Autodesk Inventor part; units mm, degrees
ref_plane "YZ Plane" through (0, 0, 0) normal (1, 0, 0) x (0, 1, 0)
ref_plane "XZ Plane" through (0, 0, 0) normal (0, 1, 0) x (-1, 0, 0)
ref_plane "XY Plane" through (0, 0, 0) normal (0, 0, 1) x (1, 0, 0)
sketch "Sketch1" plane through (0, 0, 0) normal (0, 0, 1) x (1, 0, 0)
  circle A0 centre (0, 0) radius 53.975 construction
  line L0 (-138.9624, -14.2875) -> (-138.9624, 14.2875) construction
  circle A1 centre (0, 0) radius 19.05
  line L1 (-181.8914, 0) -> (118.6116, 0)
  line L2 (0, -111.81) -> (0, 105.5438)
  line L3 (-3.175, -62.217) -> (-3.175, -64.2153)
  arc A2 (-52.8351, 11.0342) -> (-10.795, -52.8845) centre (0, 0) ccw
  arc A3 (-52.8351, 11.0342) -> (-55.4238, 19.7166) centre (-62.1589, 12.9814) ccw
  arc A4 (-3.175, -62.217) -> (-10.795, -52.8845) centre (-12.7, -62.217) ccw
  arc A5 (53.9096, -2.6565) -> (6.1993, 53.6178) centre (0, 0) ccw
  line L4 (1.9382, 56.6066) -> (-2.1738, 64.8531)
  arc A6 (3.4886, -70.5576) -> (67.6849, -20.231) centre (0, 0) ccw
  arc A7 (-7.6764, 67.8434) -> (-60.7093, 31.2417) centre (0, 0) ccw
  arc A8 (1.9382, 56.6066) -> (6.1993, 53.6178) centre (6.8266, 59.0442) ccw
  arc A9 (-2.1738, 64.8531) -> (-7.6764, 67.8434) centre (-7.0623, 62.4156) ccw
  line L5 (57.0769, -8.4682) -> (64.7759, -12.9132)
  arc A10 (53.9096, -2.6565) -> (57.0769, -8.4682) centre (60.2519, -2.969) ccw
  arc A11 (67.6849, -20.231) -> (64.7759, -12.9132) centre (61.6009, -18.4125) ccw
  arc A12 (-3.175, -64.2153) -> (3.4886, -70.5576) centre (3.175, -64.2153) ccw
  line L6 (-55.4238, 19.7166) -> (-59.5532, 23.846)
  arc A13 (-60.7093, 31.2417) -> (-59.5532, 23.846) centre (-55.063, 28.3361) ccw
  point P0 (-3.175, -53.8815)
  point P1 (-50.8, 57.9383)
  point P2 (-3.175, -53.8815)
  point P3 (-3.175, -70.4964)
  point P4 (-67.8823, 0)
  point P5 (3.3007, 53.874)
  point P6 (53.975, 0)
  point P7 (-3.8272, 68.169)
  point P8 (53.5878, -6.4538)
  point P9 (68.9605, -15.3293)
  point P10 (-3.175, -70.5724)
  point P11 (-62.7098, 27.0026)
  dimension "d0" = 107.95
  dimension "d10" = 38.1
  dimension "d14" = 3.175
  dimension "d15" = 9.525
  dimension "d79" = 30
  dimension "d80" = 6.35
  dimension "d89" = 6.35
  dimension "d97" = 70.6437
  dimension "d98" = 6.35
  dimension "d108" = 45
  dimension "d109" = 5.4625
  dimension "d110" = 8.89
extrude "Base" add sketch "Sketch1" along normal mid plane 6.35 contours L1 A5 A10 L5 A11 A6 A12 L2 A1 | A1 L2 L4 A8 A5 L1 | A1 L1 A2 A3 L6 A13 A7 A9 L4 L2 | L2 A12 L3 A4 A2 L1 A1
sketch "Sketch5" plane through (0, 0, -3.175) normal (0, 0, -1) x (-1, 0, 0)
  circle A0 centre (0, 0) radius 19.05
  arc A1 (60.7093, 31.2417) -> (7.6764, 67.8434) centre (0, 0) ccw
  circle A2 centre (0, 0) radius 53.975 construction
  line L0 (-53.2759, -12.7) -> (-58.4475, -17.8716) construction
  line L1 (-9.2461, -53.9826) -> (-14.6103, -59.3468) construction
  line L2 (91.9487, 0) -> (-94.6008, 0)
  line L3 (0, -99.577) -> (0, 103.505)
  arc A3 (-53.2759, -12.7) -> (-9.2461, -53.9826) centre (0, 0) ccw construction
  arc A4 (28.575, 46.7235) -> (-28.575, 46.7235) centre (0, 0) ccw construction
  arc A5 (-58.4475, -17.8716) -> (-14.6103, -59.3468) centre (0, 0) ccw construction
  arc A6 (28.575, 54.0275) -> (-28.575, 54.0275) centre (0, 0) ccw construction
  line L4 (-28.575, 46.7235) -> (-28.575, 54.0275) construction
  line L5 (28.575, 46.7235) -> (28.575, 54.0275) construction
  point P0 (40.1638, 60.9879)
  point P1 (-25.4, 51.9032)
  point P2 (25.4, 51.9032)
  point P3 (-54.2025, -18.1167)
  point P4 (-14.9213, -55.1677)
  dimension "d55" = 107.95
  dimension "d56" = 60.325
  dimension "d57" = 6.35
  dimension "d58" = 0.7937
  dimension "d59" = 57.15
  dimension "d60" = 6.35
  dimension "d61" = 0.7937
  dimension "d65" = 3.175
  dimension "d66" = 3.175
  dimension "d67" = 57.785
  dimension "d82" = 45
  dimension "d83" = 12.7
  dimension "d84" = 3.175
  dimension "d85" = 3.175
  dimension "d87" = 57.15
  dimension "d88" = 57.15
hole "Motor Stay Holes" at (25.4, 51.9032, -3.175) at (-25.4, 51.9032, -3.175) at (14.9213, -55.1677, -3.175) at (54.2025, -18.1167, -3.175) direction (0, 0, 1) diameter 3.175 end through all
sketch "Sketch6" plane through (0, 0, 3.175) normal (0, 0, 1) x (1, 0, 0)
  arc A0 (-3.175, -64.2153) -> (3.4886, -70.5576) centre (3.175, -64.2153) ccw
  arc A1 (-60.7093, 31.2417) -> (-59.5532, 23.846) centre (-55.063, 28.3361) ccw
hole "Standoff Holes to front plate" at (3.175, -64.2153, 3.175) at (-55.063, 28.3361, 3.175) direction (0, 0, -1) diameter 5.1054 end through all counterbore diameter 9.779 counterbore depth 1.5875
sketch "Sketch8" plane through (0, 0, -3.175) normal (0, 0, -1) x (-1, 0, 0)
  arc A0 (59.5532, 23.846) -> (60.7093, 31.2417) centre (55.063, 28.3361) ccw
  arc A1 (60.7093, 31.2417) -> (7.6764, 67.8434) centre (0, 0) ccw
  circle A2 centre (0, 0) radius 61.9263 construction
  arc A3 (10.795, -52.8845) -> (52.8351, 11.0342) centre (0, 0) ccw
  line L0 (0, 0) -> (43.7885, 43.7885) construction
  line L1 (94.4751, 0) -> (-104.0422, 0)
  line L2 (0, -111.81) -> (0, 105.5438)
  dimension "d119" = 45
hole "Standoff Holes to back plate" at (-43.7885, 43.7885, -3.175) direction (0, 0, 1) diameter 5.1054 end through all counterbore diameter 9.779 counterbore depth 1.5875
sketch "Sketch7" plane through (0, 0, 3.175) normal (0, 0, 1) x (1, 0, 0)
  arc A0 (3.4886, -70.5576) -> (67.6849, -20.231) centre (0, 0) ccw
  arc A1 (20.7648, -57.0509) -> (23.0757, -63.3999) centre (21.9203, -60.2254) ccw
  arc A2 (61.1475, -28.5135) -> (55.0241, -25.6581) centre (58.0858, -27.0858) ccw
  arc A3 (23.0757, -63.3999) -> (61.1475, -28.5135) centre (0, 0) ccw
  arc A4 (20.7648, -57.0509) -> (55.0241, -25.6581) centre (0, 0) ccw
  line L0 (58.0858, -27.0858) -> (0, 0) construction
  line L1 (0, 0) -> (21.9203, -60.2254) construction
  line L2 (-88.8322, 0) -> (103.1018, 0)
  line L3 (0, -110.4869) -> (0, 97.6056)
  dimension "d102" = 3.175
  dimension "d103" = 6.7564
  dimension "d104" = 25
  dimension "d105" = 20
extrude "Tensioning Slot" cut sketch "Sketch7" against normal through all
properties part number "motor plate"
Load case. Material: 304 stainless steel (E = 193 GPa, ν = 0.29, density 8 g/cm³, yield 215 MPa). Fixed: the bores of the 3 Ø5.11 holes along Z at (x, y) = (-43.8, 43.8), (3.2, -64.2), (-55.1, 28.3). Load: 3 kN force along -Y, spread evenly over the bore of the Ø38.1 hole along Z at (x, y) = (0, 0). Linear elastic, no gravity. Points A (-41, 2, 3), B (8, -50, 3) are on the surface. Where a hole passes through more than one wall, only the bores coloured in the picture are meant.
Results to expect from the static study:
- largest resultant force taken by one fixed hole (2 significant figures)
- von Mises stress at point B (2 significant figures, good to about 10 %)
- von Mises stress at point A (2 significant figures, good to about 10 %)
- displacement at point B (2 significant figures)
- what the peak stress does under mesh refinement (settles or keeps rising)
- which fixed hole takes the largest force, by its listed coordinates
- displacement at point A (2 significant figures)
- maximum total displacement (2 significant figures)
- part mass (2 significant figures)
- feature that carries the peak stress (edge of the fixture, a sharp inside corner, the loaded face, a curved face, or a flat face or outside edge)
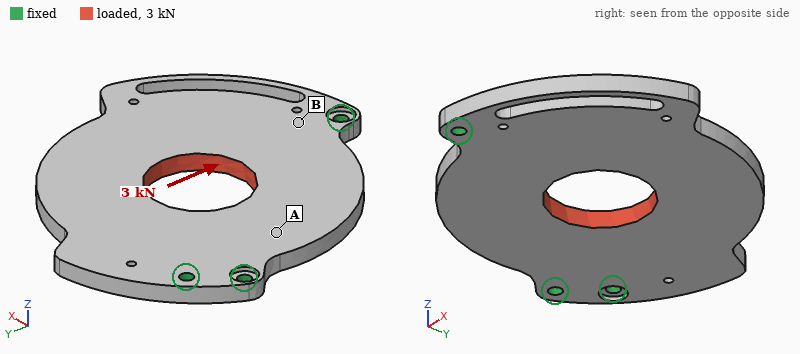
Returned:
1.7 kN
9.7 MPa
5.0 MPa
1.9 µm
keeps rising
(3.2, -64.2)
1.9 µm
6.1 µm
510 g
edge of the fixture
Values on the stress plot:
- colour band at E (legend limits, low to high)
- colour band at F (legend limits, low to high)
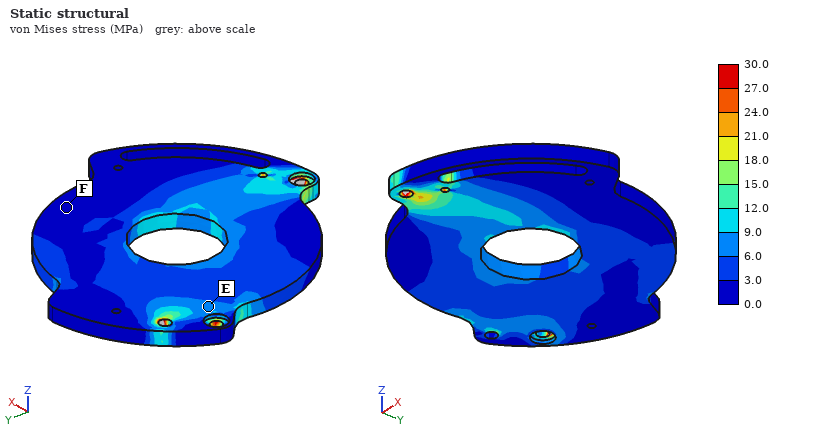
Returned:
6.0 to 9.0 MPa
0.0 to 3.0 MPa
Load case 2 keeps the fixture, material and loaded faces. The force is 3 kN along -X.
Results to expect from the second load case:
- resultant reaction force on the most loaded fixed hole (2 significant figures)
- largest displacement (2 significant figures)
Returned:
1.1 kN
4.0 µm
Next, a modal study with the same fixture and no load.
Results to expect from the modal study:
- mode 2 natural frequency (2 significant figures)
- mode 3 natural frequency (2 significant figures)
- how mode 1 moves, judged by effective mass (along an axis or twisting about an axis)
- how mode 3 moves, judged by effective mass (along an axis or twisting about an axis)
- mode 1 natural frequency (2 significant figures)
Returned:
1800 Hz
2100 Hz
along Z
along Z
650 Hz
